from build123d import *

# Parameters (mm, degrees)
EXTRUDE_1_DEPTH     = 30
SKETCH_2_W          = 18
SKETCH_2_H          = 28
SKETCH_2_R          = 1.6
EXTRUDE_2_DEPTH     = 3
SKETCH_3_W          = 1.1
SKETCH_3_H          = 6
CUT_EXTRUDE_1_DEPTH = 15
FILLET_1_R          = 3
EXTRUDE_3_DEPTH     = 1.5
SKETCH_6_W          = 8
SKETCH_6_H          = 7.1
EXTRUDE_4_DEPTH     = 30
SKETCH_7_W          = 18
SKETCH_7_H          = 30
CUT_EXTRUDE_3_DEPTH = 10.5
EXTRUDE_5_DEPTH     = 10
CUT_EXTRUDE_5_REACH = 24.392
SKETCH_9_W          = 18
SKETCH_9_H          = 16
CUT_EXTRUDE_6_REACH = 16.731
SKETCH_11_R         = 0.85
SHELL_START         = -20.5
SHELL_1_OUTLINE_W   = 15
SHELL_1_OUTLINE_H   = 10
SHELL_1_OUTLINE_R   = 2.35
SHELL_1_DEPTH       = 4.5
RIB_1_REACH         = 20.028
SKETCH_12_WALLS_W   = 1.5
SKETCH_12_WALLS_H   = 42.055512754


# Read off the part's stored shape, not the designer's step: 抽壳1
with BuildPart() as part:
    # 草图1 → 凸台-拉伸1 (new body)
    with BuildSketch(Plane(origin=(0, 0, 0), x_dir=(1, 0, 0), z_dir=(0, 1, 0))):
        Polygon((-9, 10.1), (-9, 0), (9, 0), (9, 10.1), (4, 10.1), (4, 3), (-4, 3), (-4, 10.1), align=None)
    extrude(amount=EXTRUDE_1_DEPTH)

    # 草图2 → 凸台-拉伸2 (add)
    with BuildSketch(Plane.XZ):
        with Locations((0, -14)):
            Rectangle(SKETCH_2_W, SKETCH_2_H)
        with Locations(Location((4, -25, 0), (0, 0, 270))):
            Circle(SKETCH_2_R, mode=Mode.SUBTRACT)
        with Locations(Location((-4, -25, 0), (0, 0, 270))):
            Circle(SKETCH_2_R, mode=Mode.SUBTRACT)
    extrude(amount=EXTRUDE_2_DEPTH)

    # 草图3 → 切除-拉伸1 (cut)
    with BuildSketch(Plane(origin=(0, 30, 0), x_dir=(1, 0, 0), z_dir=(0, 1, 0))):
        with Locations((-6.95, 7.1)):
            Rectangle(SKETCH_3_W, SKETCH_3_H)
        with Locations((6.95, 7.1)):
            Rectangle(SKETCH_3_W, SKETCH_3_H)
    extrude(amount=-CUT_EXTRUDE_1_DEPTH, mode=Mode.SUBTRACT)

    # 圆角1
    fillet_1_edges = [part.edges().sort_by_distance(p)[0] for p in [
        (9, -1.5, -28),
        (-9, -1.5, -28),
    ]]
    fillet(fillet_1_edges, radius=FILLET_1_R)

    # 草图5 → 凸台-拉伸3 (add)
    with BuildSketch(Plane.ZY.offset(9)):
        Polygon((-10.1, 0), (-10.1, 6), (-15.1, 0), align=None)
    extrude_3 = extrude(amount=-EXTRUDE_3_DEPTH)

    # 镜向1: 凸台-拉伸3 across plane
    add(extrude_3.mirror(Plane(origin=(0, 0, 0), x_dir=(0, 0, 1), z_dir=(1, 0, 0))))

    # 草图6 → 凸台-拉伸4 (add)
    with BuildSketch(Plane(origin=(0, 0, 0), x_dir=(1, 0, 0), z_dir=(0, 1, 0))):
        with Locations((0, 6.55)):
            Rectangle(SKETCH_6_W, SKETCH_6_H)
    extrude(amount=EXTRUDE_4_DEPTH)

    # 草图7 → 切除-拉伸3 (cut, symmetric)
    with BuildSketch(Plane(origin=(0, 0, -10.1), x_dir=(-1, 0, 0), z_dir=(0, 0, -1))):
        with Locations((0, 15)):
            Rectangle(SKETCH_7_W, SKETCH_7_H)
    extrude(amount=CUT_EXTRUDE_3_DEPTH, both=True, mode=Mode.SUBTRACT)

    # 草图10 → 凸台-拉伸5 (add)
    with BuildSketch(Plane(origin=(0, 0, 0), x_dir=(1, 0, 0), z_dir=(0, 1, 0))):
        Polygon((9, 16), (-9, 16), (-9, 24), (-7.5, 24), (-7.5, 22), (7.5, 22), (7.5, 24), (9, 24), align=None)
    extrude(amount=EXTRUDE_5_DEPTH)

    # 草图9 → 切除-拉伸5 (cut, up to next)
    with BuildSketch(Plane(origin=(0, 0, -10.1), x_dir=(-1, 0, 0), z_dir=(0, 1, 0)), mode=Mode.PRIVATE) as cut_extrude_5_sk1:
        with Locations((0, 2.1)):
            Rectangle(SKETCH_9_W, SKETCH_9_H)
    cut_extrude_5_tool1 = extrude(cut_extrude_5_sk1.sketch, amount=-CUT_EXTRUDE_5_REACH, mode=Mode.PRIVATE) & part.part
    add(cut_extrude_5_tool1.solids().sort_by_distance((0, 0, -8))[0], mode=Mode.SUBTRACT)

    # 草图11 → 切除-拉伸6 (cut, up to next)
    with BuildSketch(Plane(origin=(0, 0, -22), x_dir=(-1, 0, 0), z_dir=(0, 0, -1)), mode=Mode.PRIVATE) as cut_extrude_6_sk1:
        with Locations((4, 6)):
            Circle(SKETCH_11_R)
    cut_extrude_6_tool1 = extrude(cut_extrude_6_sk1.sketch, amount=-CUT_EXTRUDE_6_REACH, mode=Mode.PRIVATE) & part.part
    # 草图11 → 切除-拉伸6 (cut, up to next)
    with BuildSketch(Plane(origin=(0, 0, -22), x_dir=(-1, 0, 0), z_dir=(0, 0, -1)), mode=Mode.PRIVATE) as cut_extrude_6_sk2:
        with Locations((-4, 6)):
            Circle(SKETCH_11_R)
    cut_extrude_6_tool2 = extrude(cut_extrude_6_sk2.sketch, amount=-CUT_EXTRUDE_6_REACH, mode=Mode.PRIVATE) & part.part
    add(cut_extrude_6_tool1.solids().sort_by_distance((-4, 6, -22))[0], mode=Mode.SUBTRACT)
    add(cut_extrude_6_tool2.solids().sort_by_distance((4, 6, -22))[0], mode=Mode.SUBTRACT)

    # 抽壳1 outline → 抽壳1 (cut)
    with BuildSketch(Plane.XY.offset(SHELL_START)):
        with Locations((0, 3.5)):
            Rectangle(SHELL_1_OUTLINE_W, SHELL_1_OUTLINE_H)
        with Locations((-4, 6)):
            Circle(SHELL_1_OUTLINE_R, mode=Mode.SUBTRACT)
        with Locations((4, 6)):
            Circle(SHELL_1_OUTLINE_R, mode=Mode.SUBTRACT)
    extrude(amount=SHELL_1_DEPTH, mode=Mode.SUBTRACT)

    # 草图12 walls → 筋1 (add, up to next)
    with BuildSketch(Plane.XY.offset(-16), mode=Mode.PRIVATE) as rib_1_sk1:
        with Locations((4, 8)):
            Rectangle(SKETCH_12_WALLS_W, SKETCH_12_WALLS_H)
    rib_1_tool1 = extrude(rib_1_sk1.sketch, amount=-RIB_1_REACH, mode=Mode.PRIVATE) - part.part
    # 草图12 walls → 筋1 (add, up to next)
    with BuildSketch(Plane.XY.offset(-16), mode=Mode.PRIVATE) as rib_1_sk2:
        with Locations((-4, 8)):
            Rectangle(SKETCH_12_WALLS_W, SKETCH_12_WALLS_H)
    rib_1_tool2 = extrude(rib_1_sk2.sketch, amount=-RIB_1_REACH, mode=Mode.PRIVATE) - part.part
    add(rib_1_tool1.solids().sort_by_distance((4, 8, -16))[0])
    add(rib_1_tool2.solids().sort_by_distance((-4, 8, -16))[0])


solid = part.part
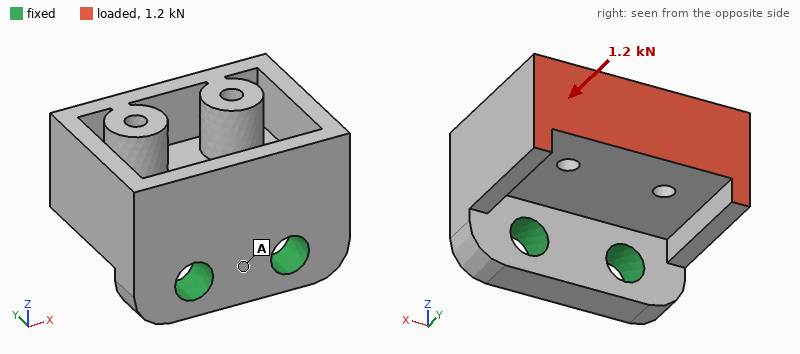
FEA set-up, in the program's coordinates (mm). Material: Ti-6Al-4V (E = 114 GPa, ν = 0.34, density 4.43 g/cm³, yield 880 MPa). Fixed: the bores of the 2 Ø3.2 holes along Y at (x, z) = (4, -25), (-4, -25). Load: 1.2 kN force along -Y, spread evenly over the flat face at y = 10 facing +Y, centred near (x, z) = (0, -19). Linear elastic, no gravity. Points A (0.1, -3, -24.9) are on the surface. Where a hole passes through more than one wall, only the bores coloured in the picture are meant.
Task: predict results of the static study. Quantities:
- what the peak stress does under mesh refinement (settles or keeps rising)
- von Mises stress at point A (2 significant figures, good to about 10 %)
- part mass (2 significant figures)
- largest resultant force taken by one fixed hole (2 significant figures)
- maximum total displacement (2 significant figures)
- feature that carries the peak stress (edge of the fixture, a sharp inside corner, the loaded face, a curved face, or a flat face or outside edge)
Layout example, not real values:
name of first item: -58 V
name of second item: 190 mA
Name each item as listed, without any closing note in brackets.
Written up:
what the peak stress does under mesh refinement: keeps rising
von Mises stress at point A: 54 MPa
part mass: 5.2 g
largest resultant force taken by one fixed hole: 600 N
maximum total displacement: 74 µm
feature that carries the peak stress: edge of the fixture
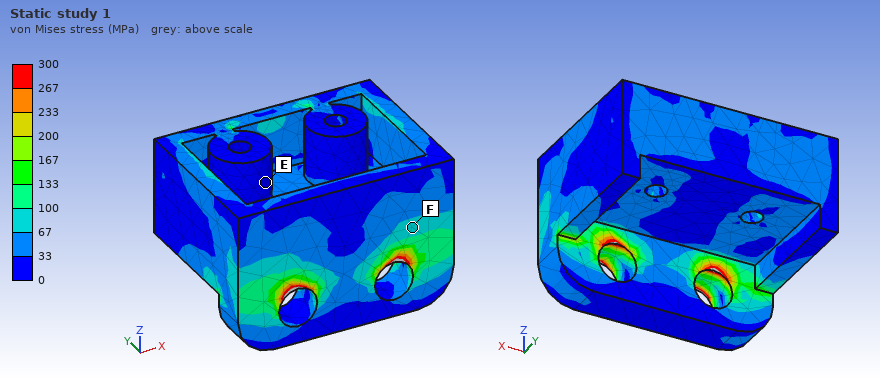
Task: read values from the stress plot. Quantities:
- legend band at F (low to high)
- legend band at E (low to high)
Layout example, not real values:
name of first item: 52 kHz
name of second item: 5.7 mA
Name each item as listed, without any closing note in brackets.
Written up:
legend band at F: 67 to 100 MPa
legend band at E: 0 to 33 MPa
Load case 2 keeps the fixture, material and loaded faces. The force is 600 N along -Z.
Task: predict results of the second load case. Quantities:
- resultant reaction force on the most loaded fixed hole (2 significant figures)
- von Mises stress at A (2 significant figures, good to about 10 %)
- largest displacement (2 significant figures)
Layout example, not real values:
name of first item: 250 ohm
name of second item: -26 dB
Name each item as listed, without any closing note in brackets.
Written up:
resultant reaction force on the most loaded fixed hole: 300 N
von Mises stress at A: 59 MPa
largest displacement: 0.12 mm
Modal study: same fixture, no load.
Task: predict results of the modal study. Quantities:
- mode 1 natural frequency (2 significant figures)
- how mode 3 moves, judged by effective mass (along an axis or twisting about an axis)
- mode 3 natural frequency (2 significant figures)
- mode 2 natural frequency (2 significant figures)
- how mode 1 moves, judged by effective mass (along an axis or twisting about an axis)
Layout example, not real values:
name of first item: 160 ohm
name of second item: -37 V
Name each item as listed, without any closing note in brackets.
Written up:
mode 1 natural frequency: 9900 Hz
how mode 3 moves, judged by effective mass: along X
mode 3 natural frequency: 22 kHz
mode 2 natural frequency: 16 kHz
how mode 1 moves, judged by effective mass: along Z
